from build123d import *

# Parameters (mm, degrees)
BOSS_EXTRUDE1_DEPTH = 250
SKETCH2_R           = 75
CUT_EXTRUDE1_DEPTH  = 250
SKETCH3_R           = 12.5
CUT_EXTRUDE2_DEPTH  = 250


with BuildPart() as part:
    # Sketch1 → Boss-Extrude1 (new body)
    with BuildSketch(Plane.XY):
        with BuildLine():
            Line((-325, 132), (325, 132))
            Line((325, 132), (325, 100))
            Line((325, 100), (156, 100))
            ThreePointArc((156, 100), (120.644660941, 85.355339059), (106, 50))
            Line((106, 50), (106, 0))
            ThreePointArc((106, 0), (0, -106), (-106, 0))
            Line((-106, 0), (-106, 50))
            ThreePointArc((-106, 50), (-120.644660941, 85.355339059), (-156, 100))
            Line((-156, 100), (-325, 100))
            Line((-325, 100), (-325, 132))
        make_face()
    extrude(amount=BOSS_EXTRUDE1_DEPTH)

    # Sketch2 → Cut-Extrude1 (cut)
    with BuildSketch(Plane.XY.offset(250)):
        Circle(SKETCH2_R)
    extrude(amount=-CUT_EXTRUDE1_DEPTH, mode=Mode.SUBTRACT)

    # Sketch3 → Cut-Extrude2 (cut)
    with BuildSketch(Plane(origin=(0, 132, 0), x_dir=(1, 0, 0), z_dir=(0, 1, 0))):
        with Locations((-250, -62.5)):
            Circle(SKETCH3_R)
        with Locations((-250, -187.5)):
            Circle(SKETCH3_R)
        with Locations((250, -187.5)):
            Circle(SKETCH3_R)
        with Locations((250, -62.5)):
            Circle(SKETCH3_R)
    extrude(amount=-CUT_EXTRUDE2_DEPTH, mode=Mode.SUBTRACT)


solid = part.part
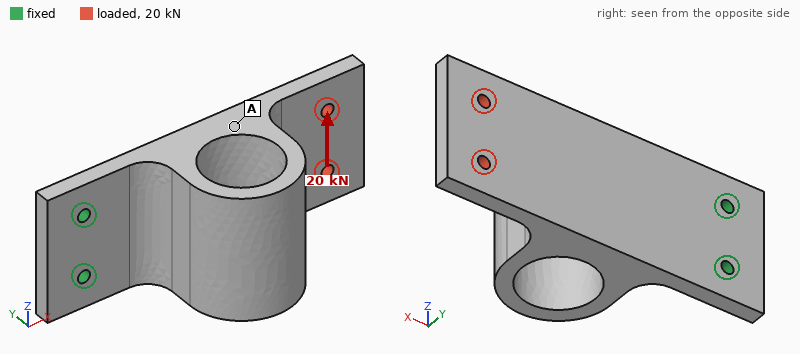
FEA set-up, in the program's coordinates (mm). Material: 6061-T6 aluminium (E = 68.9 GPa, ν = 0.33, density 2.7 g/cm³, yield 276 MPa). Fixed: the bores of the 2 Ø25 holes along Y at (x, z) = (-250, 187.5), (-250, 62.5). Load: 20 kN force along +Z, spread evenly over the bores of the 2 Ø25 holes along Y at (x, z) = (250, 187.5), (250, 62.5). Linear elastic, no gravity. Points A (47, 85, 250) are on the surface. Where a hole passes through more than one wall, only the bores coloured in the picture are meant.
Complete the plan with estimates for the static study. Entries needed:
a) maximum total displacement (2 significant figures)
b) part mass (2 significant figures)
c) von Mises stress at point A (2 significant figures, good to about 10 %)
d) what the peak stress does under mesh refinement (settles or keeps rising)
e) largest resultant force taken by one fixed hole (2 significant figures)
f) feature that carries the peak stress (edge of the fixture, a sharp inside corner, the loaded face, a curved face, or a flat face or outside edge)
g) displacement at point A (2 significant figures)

0.47 mm
29 kg
5.2 MPa
keeps rising
73 kN
edge of the fixture
0.21 mm
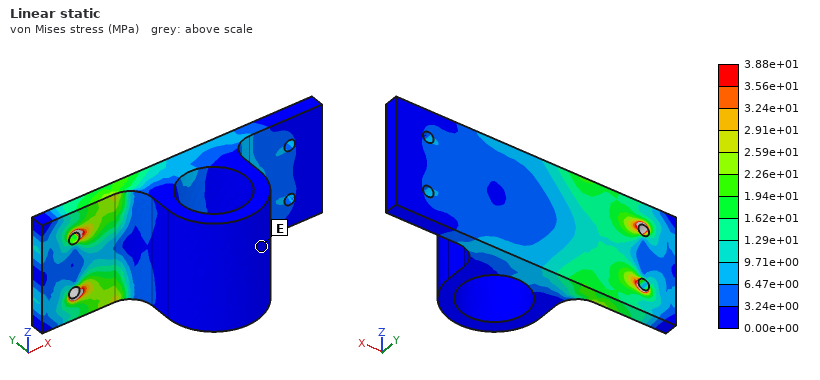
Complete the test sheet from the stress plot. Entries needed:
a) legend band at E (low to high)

0.00e+00 to 3.24e+00 MPa
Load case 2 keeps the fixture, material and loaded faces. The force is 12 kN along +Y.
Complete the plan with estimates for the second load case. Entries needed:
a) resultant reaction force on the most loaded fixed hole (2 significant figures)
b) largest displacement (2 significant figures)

6.1 kN
7.8 mm
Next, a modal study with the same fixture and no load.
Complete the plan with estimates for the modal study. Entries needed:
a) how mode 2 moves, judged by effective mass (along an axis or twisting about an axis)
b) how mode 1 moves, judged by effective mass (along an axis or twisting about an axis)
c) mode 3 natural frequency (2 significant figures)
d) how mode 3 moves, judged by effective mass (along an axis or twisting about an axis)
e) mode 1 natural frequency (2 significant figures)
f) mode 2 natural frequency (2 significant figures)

along Z
along Y
430 Hz
along Z
72 Hz
290 Hz
